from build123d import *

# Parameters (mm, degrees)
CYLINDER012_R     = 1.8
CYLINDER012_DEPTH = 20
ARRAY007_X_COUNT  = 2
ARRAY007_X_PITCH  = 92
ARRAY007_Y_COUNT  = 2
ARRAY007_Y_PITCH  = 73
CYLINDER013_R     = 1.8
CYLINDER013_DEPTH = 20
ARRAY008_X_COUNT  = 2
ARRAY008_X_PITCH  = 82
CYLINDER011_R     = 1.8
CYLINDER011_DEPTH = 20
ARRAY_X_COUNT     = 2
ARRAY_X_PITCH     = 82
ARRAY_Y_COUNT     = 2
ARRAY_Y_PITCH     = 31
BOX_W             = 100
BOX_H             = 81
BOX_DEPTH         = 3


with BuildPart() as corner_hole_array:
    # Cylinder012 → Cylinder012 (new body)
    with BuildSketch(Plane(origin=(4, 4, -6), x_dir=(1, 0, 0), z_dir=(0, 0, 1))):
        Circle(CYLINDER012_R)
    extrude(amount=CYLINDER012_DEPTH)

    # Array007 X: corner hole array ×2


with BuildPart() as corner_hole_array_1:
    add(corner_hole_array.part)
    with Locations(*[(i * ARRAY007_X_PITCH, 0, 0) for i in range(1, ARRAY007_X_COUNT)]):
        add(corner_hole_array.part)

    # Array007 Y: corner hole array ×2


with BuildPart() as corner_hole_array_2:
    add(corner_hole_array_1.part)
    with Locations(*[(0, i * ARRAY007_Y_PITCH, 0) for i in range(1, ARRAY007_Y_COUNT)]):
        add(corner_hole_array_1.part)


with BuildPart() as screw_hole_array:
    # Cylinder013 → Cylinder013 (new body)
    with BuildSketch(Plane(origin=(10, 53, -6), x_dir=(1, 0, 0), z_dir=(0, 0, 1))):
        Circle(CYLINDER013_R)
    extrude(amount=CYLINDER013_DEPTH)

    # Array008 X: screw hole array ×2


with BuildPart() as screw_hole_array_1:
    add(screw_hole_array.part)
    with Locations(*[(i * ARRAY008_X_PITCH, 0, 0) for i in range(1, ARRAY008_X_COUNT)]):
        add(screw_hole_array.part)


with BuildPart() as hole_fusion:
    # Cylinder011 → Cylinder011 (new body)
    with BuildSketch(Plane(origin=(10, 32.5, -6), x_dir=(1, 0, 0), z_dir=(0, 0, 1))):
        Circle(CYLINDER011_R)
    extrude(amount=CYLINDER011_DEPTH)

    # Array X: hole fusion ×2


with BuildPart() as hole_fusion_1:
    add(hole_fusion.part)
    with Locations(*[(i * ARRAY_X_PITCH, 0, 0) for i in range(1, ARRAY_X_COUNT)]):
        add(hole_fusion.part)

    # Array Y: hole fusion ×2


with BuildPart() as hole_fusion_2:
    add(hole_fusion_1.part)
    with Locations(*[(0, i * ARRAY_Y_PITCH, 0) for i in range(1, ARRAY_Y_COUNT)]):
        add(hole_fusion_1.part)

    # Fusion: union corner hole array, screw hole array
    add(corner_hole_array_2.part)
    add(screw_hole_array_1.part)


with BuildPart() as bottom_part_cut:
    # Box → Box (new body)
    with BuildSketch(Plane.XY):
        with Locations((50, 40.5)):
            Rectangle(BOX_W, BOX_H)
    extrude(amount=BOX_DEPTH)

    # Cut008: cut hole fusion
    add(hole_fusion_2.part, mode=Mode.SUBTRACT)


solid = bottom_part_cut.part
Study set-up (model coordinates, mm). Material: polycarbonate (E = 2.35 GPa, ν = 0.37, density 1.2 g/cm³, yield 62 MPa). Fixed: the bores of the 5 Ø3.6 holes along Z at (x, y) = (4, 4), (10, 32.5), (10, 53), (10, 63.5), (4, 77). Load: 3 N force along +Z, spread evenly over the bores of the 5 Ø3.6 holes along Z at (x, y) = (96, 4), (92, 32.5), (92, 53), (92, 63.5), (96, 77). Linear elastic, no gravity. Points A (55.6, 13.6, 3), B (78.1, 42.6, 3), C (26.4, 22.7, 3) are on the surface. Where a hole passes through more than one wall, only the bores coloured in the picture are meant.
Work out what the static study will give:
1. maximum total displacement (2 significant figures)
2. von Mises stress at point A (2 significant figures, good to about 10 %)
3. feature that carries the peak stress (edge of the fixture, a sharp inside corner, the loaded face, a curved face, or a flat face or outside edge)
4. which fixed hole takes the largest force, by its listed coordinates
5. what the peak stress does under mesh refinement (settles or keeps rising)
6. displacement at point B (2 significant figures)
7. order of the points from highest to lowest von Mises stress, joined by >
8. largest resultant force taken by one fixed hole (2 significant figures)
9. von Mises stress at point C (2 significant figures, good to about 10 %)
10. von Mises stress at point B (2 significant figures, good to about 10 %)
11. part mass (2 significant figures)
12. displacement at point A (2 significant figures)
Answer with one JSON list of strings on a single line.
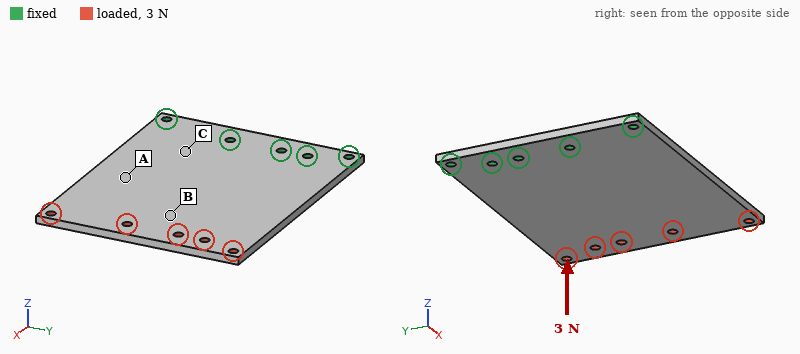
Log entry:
["1.5 mm", "0.87 MPa", "edge of the fixture", "(10, 63.5)", "keeps rising", "0.96 mm", "C > A > B", "3.2 N", "1.4 MPa", "0.37 MPa", "29 g", "0.48 mm"]
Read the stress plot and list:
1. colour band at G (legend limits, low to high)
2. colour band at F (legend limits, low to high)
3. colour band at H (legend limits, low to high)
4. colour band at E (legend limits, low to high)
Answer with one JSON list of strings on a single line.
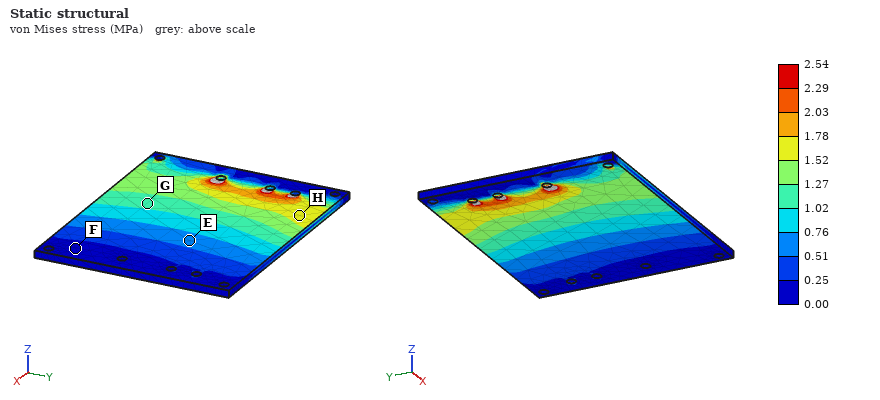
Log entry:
["1.02 to 1.27 MPa", "0.00 to 0.25 MPa", "1.52 to 1.78 MPa", "0.51 to 0.76 MPa"]
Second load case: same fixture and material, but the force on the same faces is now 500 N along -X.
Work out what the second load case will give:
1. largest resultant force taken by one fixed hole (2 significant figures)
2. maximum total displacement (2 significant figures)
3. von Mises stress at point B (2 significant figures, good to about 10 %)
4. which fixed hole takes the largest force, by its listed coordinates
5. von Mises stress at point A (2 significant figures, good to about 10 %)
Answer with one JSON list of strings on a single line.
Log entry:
["130 N", "0.13 mm", "1.7 MPa", "(10, 32.5)", "1.5 MPa"]
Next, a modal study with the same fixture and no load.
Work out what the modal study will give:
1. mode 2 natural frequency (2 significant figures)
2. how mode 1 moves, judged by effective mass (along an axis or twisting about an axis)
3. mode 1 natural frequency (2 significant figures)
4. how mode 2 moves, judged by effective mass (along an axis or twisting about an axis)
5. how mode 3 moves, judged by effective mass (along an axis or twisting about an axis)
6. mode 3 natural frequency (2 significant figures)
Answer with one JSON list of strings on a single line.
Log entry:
["210 Hz", "along Z", "86 Hz", "twisting about X", "along Z", "510 Hz"]
